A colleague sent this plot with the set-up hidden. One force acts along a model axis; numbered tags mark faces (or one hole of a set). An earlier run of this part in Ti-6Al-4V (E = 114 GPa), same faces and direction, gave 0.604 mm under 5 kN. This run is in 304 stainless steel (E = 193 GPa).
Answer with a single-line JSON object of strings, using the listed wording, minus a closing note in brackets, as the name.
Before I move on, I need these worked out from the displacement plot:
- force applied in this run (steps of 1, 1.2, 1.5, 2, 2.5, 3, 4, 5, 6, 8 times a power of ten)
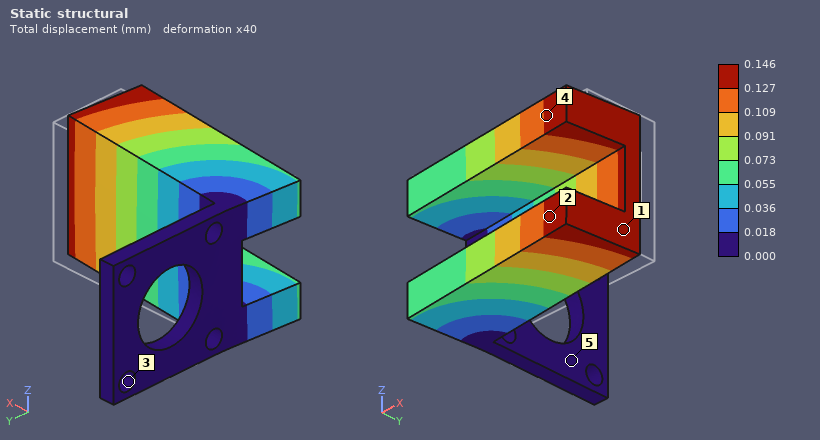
{"force applied in this run": "2 kN"}
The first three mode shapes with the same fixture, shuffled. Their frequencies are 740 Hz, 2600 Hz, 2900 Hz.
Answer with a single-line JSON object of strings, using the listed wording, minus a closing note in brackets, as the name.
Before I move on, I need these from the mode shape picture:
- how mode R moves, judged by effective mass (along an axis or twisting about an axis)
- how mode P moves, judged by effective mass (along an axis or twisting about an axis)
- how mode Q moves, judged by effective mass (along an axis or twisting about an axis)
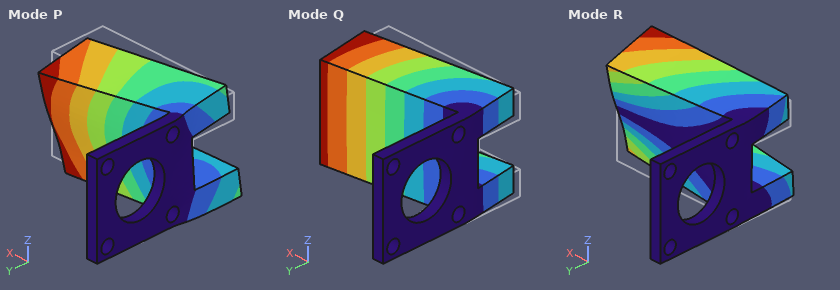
{"how mode R moves, judged by effective mass": "along Z", "how mode P moves, judged by effective mass": "along Z", "how mode Q moves, judged by effective mass": "along Y"}
